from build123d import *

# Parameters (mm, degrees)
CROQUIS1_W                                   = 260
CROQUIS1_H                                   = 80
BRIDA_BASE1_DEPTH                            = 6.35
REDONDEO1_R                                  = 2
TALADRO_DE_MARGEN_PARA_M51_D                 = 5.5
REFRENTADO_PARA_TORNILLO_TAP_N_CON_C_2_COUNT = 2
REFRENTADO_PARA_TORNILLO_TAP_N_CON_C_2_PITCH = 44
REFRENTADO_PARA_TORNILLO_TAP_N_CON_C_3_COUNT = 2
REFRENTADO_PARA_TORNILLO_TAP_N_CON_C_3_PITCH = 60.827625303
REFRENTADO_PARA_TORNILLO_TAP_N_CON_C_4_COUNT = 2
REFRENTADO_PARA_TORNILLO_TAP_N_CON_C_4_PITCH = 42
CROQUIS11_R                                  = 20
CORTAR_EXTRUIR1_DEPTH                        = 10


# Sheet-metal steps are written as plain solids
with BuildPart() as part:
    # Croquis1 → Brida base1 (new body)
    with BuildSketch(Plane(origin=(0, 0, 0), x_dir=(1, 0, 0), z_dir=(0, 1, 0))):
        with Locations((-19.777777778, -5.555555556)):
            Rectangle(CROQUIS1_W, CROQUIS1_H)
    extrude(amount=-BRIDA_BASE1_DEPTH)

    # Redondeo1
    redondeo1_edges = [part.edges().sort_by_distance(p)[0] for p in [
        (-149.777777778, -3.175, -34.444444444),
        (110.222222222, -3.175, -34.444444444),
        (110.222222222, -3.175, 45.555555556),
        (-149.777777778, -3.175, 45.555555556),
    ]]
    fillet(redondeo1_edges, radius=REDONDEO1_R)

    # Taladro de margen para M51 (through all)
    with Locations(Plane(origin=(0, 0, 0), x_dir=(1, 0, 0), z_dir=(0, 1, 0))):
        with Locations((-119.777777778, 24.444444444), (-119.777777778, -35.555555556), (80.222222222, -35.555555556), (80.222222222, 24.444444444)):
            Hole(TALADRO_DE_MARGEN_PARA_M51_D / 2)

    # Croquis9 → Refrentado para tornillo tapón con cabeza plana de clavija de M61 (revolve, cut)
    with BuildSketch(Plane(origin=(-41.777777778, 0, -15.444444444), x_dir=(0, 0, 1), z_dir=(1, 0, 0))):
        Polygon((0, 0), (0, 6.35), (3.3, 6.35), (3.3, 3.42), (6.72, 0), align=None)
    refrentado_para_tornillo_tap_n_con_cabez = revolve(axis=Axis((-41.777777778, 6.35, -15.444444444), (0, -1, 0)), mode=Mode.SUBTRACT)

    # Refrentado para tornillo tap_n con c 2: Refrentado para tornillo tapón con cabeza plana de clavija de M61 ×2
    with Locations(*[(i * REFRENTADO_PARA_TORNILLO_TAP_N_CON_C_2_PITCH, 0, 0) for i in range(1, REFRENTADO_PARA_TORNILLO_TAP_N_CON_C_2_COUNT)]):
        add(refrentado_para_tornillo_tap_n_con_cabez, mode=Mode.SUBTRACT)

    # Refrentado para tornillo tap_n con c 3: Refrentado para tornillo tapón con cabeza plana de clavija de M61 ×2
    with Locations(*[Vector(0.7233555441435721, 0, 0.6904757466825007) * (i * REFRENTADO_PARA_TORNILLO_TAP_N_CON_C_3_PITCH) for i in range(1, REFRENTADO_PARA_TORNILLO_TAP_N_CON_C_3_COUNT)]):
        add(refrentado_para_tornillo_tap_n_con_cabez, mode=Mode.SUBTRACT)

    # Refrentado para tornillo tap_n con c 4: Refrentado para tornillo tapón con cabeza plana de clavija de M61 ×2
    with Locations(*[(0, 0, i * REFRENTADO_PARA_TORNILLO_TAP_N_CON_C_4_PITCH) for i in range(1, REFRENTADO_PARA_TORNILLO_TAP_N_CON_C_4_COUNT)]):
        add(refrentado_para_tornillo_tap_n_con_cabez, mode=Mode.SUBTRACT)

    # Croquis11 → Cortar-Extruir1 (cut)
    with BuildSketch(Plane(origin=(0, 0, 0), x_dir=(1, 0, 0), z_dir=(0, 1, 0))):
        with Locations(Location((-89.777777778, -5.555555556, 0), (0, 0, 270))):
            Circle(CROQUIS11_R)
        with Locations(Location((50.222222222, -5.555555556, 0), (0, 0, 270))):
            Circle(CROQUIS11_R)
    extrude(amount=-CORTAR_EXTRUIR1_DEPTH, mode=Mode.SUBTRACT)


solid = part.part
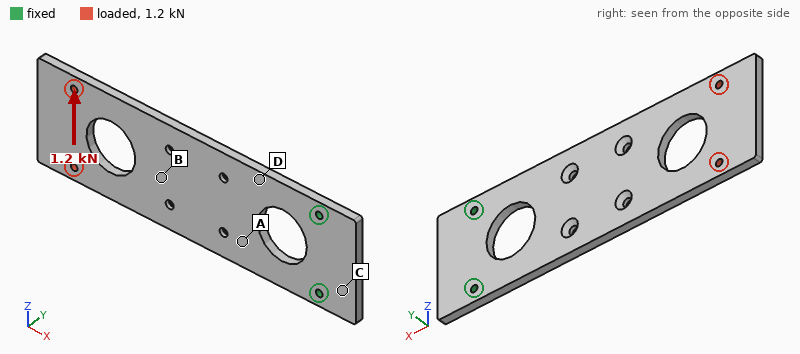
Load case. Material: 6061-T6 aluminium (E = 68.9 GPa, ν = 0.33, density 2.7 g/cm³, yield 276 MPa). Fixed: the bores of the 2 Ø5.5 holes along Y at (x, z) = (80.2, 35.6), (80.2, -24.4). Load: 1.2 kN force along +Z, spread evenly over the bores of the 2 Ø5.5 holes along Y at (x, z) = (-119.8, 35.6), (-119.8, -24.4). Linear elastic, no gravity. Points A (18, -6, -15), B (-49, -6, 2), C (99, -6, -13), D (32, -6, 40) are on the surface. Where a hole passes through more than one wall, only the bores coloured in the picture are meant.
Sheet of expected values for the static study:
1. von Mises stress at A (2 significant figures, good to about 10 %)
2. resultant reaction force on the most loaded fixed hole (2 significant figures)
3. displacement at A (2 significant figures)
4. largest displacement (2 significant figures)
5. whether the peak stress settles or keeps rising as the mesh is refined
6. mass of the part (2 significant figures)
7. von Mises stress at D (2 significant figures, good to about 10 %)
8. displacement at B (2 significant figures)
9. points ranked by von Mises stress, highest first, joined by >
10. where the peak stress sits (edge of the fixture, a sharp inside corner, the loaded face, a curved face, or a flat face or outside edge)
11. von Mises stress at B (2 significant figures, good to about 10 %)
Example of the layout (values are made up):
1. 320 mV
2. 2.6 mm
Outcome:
1. 14 MPa
2. 3.9 kN
3. 0.052 mm
4. 0.30 mm
5. keeps rising
6. 310 g
7. 21 MPa
8. 0.13 mm
9. D > A > B > C
10. edge of the fixture
11. 10 MPa
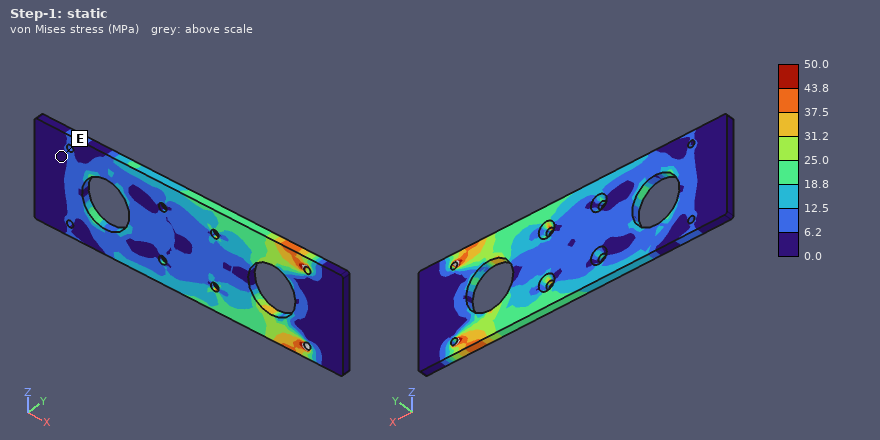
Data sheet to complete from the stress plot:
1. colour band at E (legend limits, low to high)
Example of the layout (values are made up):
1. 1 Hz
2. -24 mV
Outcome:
1. 0.0 to 6.2 MPa
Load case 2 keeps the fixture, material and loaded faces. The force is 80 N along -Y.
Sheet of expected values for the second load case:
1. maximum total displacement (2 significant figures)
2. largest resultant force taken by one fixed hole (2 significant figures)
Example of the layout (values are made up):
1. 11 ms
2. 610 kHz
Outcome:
1. 3.2 mm
2. 40 N
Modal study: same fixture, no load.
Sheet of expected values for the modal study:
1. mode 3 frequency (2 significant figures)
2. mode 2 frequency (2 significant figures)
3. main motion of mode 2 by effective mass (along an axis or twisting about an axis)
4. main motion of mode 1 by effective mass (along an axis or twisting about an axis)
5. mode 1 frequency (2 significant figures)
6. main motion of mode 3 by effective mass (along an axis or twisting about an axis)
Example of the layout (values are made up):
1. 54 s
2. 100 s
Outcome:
1. 550 Hz
2. 520 Hz
3. twisting about X
4. along Y
5. 86 Hz
6. along Y
